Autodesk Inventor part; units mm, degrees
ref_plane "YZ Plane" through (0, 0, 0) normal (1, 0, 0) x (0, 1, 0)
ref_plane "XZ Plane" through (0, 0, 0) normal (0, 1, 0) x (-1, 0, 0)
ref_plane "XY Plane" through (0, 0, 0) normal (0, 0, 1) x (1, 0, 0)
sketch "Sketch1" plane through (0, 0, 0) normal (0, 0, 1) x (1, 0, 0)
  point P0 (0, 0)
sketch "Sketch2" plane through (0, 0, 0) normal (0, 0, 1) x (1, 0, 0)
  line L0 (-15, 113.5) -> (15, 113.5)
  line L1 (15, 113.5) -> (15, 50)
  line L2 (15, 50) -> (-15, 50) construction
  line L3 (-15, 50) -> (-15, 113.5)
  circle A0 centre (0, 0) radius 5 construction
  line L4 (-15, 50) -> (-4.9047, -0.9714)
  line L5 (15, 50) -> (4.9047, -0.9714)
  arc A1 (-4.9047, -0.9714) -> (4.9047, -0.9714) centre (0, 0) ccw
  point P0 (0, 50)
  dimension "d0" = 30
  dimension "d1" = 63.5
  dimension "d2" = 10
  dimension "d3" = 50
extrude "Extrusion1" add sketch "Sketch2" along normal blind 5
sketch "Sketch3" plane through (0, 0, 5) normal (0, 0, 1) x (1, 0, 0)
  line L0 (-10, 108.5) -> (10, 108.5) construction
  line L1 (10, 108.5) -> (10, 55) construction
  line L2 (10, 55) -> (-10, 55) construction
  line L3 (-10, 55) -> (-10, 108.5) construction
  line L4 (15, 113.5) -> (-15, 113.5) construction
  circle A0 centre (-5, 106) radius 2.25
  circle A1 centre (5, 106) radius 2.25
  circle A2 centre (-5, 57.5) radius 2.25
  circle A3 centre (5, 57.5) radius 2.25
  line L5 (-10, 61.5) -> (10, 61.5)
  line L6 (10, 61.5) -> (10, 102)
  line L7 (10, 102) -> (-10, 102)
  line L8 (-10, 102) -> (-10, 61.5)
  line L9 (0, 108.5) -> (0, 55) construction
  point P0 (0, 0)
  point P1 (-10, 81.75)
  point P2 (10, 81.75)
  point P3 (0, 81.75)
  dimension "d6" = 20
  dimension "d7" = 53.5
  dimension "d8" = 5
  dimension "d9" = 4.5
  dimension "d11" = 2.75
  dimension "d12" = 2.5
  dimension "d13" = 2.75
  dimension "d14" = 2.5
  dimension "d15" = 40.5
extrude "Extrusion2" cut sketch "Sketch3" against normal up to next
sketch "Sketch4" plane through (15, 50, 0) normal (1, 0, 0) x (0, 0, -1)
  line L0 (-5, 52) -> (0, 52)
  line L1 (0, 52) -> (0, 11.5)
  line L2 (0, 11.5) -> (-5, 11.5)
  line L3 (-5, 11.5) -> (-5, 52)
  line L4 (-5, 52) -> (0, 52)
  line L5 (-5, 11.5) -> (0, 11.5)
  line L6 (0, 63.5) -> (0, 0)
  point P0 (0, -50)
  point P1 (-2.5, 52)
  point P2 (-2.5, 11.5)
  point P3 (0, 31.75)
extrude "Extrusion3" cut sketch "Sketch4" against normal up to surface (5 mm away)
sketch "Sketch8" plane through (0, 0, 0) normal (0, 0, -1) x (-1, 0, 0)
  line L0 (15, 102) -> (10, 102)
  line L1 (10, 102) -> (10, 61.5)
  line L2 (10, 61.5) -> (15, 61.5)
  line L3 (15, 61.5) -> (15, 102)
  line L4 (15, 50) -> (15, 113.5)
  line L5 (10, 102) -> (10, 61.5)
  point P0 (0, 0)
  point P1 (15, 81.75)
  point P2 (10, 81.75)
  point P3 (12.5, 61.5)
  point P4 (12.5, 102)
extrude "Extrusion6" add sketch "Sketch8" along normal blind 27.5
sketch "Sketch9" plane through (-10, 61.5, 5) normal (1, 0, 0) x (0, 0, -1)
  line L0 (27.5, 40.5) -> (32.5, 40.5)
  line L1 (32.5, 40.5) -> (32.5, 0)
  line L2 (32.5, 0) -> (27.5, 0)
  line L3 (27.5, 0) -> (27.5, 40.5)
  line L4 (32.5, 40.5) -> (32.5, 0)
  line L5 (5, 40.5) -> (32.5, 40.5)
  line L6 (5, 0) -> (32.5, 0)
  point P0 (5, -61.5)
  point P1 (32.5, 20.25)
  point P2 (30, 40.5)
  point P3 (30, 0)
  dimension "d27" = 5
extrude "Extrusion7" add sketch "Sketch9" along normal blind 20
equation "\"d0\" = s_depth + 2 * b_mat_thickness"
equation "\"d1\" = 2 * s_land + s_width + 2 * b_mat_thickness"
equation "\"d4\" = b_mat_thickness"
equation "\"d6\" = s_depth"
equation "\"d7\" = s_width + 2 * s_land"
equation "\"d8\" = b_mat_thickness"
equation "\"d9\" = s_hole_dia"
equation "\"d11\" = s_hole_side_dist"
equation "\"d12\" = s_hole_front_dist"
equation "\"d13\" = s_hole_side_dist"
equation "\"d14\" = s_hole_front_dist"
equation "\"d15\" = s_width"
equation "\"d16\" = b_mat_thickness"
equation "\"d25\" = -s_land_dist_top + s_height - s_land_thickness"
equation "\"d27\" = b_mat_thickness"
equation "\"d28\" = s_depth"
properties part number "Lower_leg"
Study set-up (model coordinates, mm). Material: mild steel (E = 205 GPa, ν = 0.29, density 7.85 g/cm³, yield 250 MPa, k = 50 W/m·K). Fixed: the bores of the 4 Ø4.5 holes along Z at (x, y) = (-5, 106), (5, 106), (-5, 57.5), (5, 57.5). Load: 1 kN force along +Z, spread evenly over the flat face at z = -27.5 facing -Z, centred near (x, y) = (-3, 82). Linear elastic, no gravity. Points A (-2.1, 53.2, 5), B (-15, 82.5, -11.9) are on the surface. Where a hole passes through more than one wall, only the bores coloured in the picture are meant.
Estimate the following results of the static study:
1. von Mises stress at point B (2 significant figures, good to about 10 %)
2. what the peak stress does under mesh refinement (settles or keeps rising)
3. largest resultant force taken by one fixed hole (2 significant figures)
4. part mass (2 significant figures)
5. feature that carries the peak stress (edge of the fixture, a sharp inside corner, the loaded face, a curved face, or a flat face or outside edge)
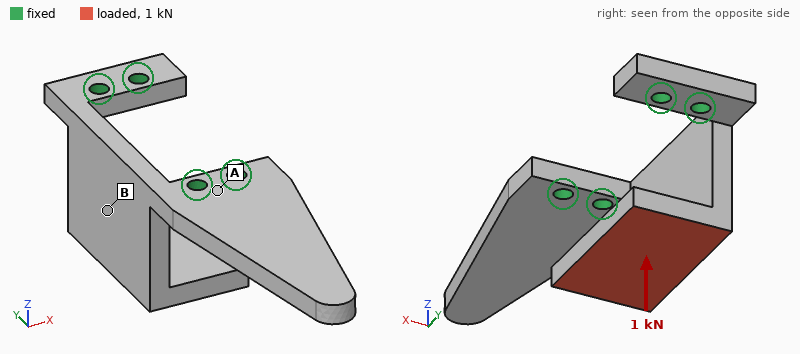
48 MPa
keeps rising
510 N
150 g
a sharp inside corner
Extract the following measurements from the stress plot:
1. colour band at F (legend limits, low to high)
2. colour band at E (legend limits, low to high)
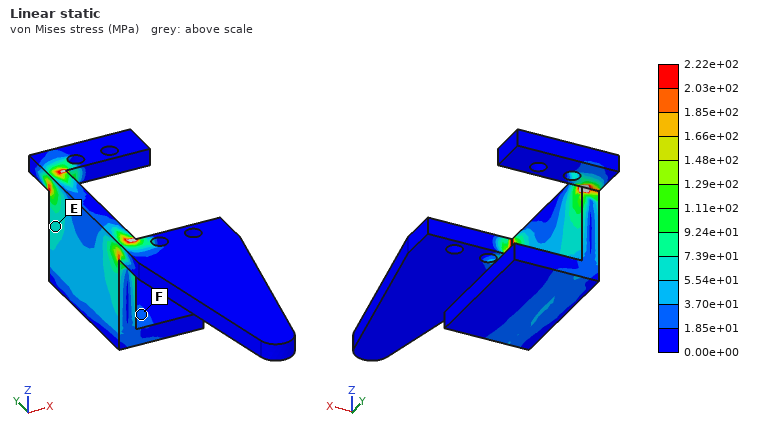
1.85e+01 to 3.70e+01 MPa
5.54e+01 to 7.39e+01 MPa
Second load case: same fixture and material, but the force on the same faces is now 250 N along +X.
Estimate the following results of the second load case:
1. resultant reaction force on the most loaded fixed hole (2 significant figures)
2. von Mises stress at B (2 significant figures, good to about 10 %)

150 N
20 MPa
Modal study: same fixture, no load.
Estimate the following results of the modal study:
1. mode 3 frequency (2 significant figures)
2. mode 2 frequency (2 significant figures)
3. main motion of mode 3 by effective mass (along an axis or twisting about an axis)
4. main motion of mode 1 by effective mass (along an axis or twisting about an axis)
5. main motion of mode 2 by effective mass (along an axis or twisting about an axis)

3300 Hz
1600 Hz
along Y
along X
along Z
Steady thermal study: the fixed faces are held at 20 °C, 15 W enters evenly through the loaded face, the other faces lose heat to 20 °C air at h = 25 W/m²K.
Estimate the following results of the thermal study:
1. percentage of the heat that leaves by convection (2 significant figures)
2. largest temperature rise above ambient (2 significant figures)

37 %
73 K
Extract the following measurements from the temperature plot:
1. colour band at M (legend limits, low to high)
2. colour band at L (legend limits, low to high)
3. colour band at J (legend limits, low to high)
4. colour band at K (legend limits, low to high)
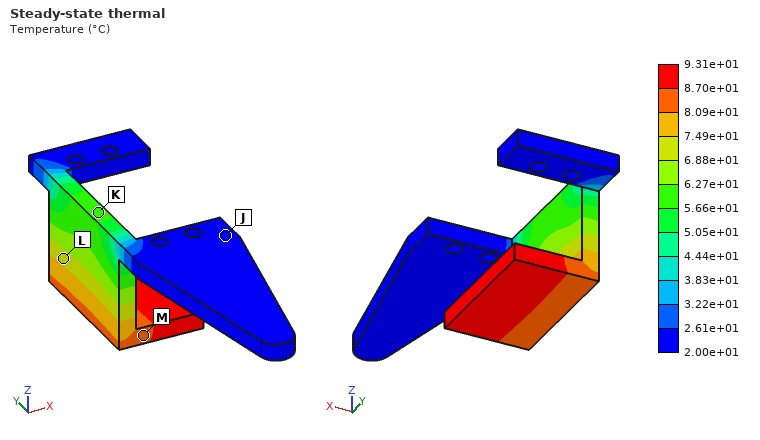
8.09e+01 to 8.70e+01 °C
6.88e+01 to 7.49e+01 °C
2.00e+01 to 2.61e+01 °C
5.66e+01 to 6.27e+01 °C
